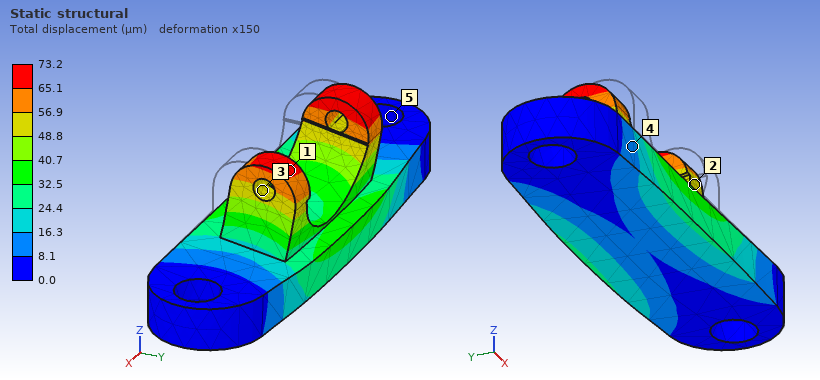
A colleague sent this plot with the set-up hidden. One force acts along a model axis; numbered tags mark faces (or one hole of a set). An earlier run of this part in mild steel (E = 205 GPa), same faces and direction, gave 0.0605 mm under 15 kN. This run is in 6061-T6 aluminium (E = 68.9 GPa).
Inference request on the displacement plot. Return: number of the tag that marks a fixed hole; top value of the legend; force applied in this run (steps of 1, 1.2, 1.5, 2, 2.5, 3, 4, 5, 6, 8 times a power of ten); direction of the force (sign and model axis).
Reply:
5
73.2 µm
6 kN
+Y
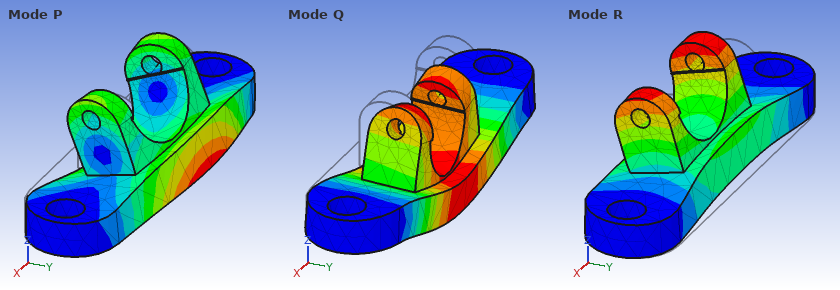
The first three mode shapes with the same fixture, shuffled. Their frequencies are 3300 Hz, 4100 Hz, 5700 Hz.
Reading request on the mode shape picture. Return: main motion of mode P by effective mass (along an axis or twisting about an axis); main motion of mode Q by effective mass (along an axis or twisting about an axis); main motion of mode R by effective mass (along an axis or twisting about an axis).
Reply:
along Y
along Z
along Y
